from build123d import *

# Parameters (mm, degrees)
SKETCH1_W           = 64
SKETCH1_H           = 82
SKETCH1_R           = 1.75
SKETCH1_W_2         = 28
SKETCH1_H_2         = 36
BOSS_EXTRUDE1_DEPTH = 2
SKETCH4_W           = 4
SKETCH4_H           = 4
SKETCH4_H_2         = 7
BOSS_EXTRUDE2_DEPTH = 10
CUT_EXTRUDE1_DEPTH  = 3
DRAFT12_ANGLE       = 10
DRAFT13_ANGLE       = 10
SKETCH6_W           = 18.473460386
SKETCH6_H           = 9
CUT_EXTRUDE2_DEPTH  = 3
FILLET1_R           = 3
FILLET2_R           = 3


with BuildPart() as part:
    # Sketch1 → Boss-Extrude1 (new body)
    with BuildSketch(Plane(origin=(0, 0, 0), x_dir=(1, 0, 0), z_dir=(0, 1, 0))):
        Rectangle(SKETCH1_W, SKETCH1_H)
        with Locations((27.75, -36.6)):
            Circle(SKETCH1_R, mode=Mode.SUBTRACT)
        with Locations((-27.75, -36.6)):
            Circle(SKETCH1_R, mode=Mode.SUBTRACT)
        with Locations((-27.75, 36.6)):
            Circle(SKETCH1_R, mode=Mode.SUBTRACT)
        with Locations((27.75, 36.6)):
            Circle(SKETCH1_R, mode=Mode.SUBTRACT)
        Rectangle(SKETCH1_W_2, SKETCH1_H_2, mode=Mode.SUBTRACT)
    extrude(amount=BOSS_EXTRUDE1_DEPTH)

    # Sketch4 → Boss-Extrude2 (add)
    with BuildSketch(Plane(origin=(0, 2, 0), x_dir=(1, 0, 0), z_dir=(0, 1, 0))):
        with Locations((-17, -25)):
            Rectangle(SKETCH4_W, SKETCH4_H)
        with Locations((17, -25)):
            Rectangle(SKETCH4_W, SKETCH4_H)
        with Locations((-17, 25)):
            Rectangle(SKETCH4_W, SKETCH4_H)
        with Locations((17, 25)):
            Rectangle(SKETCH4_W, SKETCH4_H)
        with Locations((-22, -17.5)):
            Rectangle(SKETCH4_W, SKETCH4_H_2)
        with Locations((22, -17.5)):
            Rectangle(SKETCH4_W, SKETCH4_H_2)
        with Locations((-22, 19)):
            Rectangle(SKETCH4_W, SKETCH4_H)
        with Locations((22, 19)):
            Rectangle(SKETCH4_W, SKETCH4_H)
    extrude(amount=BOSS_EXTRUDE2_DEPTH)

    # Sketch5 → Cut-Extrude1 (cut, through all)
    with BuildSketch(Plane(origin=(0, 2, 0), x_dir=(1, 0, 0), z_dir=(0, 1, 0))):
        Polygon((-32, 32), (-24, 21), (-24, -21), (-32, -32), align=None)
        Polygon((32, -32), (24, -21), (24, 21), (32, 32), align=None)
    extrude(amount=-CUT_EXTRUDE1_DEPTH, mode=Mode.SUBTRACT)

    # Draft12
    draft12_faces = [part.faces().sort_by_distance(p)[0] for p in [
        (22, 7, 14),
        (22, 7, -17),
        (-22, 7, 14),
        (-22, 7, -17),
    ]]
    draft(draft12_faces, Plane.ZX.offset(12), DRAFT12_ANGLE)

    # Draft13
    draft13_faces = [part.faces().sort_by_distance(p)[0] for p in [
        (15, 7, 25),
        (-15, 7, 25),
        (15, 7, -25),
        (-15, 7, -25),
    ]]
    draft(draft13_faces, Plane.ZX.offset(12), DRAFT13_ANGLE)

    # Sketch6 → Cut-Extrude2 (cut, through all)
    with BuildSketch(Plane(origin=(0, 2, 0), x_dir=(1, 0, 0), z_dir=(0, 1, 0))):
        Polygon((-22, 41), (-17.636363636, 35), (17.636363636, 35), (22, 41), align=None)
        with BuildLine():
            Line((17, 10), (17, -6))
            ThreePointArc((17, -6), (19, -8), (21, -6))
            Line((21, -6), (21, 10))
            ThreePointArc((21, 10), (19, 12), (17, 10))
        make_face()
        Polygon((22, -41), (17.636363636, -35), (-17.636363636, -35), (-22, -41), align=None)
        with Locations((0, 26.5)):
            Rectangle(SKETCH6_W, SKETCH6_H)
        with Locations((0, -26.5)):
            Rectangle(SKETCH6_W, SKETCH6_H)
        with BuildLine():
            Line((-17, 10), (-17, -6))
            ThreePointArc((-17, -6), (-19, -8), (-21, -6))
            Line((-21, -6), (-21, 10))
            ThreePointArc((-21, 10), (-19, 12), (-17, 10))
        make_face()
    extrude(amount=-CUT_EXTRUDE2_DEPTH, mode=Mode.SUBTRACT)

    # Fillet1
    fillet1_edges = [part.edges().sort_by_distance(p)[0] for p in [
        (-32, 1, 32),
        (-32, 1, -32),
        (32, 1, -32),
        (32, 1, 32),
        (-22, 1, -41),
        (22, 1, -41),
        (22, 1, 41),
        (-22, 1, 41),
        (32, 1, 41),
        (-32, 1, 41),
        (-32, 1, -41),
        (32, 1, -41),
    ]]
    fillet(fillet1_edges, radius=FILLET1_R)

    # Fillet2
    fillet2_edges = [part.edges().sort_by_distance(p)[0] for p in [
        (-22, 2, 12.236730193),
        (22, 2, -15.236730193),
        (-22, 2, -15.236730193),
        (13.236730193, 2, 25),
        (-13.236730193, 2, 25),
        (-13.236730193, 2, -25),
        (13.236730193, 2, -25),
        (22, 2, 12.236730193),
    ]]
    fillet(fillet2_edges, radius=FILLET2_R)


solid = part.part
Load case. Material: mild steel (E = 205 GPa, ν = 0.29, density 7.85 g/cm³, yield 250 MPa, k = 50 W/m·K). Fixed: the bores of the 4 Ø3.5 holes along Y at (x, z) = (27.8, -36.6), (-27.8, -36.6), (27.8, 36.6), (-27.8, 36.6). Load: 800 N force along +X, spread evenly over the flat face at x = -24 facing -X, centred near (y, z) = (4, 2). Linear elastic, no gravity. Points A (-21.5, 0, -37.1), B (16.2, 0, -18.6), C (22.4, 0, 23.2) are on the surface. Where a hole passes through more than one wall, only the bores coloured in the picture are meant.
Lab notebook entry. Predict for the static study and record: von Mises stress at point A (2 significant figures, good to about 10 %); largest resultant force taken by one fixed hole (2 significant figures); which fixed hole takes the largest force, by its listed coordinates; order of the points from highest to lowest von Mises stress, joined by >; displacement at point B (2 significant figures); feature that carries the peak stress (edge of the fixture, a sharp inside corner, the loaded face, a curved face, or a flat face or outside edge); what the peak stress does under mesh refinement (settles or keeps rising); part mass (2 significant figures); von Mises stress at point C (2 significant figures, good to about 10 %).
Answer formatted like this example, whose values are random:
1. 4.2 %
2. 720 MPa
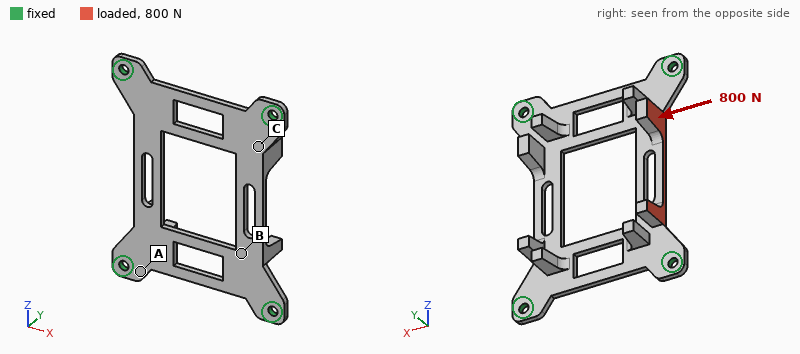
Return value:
1. 43 MPa
2. 360 N
3. (-27.8, 36.6)
4. A > C > B
5. 23 µm
6. a sharp inside corner
7. keeps rising
8. 52 g
9. 29 MPa
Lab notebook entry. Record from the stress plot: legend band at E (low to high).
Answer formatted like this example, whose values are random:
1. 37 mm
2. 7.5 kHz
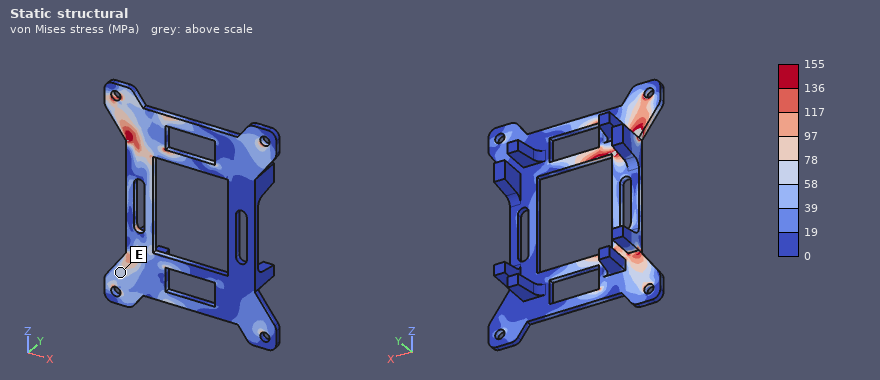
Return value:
1. 58 to 78 MPa
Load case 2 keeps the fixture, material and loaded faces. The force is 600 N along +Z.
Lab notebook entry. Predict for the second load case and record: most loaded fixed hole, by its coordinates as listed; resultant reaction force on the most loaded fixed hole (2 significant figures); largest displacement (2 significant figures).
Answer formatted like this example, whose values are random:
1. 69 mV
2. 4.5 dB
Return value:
1. (-27.8, 36.6)
2. 310 N
3. 39 µm
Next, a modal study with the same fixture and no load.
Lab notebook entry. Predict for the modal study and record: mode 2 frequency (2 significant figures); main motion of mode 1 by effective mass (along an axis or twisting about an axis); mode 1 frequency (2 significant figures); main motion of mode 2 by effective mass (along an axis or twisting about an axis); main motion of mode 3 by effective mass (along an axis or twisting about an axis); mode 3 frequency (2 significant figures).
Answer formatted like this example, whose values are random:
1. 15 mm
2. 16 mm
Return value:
1. 2200 Hz
2. along Y
3. 1600 Hz
4. twisting about Z
5. twisting about X
6. 2900 Hz
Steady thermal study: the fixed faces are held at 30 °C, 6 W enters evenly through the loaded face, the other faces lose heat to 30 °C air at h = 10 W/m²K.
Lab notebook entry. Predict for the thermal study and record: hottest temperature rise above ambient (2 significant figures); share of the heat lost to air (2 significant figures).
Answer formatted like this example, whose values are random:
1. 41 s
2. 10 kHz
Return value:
1. 52 K
2. 16 %
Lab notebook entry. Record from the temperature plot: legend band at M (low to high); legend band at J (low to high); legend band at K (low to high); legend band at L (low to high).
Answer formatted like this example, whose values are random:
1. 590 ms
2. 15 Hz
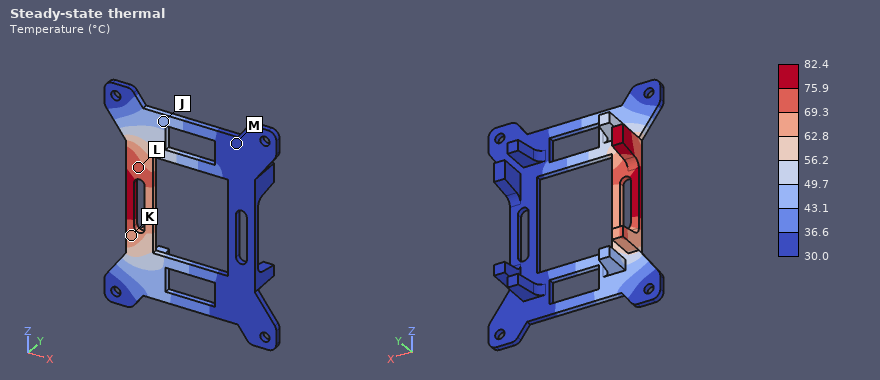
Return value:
1. 30.0 to 36.6 °C
2. 43.1 to 49.7 °C
3. 62.8 to 69.3 °C
4. 69.3 to 75.9 °C
